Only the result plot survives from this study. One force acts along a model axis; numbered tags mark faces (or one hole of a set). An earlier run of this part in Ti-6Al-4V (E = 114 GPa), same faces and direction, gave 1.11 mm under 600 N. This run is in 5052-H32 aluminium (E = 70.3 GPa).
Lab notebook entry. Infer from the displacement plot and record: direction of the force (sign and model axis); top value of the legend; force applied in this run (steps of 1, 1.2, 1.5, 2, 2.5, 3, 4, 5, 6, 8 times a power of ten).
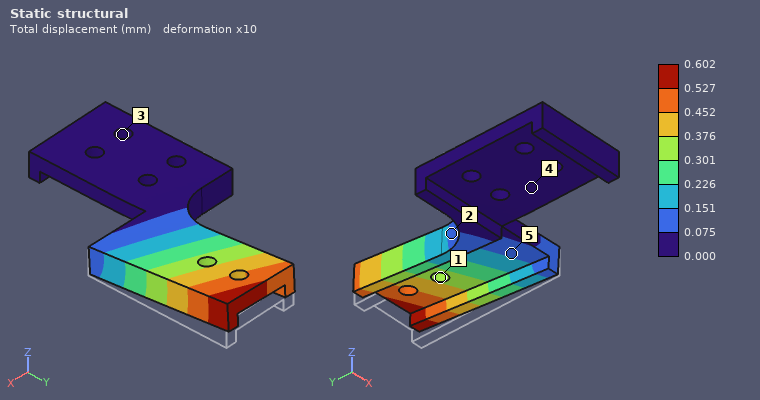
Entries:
+Z
0.602 mm
200 N
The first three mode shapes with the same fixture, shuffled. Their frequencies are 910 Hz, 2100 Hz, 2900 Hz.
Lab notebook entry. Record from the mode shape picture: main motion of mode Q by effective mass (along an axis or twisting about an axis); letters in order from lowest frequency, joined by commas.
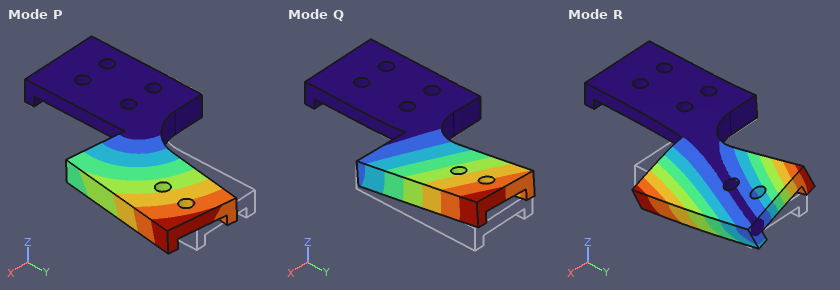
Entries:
along Z
Q, P, R
